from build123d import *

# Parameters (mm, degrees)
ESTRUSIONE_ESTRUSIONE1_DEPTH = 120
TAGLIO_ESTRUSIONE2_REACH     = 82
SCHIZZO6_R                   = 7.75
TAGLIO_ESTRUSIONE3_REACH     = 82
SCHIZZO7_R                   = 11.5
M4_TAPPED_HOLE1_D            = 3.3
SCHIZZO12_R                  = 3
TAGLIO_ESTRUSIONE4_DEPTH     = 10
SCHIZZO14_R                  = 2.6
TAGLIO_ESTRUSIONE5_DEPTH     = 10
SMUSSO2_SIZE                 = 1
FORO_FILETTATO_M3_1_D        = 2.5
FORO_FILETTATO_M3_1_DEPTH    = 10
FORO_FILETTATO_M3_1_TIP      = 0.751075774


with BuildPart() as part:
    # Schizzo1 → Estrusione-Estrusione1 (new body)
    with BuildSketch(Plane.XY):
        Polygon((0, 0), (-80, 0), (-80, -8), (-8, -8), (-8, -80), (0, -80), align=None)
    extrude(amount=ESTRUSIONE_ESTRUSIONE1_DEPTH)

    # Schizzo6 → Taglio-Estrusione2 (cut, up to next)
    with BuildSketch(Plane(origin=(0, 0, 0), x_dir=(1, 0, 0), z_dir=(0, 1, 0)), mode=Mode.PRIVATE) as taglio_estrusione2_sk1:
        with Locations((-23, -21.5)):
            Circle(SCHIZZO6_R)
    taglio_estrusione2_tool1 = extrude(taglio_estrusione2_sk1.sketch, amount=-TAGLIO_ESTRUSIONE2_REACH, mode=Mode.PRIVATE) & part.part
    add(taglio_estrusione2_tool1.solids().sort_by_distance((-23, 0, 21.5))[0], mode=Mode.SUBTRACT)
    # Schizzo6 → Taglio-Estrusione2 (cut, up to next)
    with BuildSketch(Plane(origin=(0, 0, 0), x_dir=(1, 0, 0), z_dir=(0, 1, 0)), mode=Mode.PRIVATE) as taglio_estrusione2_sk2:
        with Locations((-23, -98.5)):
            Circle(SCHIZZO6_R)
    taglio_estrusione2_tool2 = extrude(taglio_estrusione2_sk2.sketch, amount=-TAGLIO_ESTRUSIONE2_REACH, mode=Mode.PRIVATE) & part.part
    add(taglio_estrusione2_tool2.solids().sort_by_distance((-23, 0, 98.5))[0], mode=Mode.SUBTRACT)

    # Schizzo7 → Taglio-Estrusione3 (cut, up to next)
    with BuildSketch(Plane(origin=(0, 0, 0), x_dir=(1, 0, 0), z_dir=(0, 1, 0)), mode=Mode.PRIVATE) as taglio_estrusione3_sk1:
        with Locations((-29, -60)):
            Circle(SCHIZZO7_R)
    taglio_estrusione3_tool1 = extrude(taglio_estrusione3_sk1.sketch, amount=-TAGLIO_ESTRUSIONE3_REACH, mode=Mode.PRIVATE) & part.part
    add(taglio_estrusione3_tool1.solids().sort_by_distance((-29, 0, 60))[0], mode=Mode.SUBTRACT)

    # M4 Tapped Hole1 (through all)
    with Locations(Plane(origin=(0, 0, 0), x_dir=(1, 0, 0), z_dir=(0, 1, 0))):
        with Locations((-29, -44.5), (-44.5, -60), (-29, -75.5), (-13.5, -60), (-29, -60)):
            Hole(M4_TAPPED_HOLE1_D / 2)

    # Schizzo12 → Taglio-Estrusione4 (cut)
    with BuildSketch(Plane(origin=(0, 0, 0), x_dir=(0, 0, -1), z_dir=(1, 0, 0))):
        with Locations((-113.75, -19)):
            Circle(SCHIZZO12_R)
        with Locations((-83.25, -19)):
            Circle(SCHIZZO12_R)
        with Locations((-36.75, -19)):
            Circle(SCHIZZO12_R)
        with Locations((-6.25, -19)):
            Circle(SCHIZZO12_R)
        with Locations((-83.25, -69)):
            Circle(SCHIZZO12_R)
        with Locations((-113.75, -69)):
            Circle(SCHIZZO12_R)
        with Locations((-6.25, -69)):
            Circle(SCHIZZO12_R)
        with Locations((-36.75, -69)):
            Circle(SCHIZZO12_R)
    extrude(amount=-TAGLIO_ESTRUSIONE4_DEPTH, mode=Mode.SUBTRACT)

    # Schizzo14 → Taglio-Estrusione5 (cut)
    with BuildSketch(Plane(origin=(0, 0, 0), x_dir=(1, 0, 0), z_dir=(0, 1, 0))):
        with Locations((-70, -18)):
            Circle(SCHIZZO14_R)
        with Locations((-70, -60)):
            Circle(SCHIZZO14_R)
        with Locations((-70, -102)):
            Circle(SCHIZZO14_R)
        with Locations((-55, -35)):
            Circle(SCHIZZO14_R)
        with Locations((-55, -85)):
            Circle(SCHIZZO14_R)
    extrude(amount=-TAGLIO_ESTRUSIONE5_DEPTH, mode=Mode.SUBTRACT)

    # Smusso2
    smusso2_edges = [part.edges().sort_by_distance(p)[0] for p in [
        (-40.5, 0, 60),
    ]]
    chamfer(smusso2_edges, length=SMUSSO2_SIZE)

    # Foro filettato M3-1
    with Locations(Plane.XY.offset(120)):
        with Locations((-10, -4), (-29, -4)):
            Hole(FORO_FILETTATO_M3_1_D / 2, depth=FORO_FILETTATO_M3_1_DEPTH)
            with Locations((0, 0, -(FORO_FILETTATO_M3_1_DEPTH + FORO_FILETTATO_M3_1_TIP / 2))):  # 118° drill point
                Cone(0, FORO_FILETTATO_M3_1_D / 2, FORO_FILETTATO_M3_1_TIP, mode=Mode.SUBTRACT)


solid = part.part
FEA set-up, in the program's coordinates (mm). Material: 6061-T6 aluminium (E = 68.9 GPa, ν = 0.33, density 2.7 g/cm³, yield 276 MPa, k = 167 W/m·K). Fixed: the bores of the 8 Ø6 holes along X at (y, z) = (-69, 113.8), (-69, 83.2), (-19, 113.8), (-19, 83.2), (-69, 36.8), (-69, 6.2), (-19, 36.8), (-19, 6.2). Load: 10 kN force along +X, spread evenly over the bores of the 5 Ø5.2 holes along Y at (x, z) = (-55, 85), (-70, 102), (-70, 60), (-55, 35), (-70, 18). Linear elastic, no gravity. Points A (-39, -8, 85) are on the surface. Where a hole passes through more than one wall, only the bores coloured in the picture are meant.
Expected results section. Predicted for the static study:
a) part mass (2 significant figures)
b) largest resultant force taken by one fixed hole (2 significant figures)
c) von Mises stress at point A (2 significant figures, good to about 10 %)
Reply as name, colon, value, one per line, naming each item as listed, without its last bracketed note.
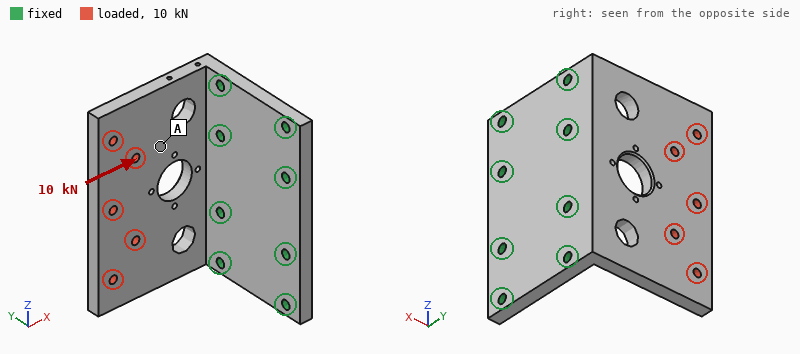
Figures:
part mass: 370 g
largest resultant force taken by one fixed hole: 3.1 kN
von Mises stress at point A: 17 MPa
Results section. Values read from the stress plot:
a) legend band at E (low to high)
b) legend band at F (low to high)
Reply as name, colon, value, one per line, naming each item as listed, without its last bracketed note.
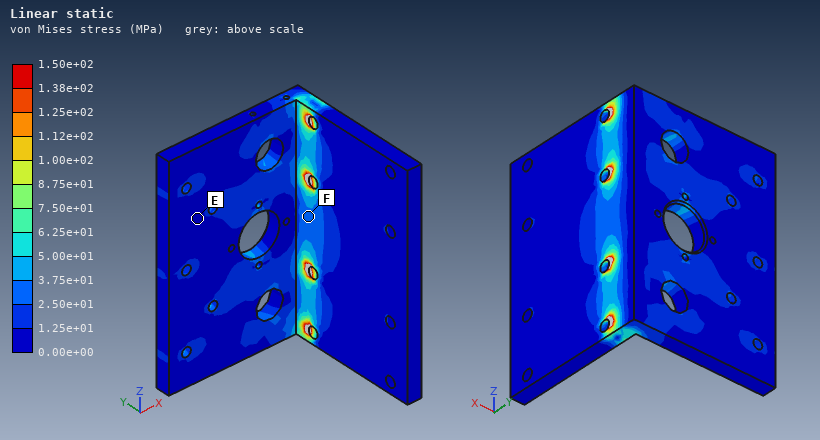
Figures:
legend band at E: 0.00e+00 to 1.25e+01 MPa
legend band at F: 2.50e+01 to 3.75e+01 MPa
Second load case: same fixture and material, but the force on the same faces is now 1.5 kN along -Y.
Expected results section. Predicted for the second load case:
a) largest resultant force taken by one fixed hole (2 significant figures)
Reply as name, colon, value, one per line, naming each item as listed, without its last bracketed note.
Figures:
largest resultant force taken by one fixed hole: 580 N
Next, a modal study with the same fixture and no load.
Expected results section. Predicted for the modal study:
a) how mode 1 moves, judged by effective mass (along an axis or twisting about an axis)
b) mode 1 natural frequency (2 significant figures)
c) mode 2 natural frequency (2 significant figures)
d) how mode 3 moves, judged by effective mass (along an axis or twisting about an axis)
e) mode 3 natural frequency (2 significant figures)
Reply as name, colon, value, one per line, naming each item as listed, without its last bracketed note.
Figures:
how mode 1 moves, judged by effective mass: along Y
mode 1 natural frequency: 820 Hz
mode 2 natural frequency: 1600 Hz
how mode 3 moves, judged by effective mass: along Z
mode 3 natural frequency: 3900 Hz
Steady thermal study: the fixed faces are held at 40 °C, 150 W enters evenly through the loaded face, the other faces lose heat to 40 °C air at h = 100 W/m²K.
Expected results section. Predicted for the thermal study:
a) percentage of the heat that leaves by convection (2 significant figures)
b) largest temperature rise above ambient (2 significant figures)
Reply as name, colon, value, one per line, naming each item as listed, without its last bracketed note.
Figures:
percentage of the heat that leaves by convection: 48 %
largest temperature rise above ambient: 57 K
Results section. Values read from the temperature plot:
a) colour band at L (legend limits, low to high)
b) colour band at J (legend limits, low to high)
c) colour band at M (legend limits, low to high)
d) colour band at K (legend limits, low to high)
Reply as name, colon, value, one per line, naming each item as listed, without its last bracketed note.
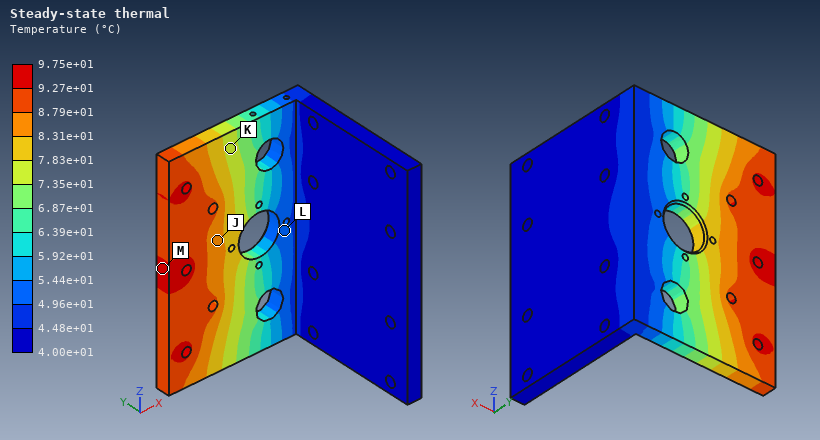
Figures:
colour band at L: 4.96e+01 to 5.44e+01 °C
colour band at J: 8.31e+01 to 8.79e+01 °C
colour band at M: 9.27e+01 to 9.75e+01 °C
colour band at K: 7.35e+01 to 7.83e+01 °C
